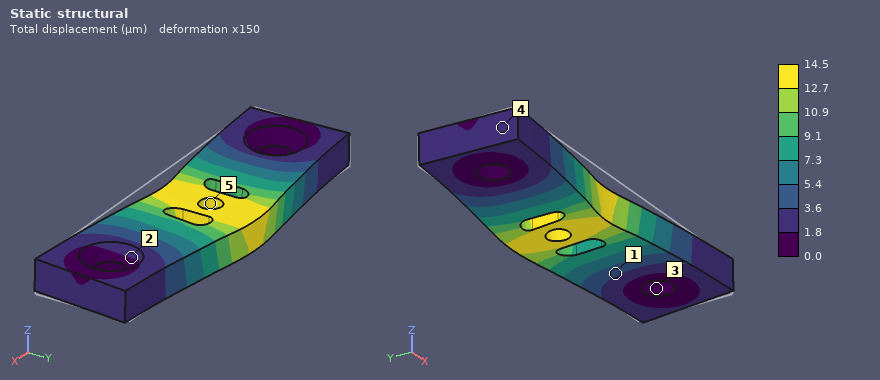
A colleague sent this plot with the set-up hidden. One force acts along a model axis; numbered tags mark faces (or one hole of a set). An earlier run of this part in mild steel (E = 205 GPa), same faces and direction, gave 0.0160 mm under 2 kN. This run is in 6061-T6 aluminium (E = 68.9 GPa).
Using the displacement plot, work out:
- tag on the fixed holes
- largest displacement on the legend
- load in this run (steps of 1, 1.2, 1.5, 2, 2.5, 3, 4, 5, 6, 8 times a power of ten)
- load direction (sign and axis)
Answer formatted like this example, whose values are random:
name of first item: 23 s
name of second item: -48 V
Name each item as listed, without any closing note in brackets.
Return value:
tag on the fixed holes: 3
largest displacement on the legend: 14.5 µm
load in this run: 600 N
load direction: +Y
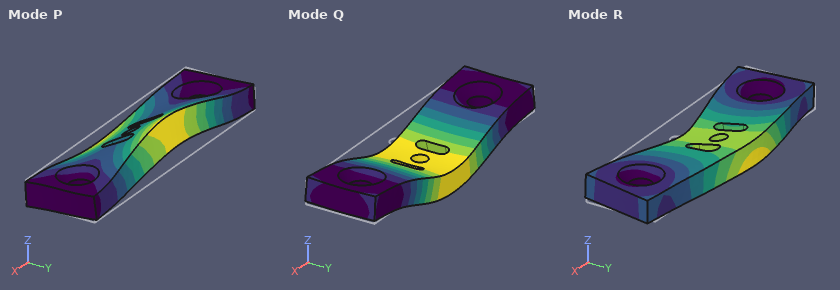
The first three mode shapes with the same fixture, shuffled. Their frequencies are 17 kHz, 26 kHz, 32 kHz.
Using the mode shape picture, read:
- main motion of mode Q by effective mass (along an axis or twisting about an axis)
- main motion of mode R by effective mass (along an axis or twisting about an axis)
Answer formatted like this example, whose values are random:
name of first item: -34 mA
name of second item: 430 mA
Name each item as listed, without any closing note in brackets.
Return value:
main motion of mode Q by effective mass: along Z
main motion of mode R by effective mass: along Y
